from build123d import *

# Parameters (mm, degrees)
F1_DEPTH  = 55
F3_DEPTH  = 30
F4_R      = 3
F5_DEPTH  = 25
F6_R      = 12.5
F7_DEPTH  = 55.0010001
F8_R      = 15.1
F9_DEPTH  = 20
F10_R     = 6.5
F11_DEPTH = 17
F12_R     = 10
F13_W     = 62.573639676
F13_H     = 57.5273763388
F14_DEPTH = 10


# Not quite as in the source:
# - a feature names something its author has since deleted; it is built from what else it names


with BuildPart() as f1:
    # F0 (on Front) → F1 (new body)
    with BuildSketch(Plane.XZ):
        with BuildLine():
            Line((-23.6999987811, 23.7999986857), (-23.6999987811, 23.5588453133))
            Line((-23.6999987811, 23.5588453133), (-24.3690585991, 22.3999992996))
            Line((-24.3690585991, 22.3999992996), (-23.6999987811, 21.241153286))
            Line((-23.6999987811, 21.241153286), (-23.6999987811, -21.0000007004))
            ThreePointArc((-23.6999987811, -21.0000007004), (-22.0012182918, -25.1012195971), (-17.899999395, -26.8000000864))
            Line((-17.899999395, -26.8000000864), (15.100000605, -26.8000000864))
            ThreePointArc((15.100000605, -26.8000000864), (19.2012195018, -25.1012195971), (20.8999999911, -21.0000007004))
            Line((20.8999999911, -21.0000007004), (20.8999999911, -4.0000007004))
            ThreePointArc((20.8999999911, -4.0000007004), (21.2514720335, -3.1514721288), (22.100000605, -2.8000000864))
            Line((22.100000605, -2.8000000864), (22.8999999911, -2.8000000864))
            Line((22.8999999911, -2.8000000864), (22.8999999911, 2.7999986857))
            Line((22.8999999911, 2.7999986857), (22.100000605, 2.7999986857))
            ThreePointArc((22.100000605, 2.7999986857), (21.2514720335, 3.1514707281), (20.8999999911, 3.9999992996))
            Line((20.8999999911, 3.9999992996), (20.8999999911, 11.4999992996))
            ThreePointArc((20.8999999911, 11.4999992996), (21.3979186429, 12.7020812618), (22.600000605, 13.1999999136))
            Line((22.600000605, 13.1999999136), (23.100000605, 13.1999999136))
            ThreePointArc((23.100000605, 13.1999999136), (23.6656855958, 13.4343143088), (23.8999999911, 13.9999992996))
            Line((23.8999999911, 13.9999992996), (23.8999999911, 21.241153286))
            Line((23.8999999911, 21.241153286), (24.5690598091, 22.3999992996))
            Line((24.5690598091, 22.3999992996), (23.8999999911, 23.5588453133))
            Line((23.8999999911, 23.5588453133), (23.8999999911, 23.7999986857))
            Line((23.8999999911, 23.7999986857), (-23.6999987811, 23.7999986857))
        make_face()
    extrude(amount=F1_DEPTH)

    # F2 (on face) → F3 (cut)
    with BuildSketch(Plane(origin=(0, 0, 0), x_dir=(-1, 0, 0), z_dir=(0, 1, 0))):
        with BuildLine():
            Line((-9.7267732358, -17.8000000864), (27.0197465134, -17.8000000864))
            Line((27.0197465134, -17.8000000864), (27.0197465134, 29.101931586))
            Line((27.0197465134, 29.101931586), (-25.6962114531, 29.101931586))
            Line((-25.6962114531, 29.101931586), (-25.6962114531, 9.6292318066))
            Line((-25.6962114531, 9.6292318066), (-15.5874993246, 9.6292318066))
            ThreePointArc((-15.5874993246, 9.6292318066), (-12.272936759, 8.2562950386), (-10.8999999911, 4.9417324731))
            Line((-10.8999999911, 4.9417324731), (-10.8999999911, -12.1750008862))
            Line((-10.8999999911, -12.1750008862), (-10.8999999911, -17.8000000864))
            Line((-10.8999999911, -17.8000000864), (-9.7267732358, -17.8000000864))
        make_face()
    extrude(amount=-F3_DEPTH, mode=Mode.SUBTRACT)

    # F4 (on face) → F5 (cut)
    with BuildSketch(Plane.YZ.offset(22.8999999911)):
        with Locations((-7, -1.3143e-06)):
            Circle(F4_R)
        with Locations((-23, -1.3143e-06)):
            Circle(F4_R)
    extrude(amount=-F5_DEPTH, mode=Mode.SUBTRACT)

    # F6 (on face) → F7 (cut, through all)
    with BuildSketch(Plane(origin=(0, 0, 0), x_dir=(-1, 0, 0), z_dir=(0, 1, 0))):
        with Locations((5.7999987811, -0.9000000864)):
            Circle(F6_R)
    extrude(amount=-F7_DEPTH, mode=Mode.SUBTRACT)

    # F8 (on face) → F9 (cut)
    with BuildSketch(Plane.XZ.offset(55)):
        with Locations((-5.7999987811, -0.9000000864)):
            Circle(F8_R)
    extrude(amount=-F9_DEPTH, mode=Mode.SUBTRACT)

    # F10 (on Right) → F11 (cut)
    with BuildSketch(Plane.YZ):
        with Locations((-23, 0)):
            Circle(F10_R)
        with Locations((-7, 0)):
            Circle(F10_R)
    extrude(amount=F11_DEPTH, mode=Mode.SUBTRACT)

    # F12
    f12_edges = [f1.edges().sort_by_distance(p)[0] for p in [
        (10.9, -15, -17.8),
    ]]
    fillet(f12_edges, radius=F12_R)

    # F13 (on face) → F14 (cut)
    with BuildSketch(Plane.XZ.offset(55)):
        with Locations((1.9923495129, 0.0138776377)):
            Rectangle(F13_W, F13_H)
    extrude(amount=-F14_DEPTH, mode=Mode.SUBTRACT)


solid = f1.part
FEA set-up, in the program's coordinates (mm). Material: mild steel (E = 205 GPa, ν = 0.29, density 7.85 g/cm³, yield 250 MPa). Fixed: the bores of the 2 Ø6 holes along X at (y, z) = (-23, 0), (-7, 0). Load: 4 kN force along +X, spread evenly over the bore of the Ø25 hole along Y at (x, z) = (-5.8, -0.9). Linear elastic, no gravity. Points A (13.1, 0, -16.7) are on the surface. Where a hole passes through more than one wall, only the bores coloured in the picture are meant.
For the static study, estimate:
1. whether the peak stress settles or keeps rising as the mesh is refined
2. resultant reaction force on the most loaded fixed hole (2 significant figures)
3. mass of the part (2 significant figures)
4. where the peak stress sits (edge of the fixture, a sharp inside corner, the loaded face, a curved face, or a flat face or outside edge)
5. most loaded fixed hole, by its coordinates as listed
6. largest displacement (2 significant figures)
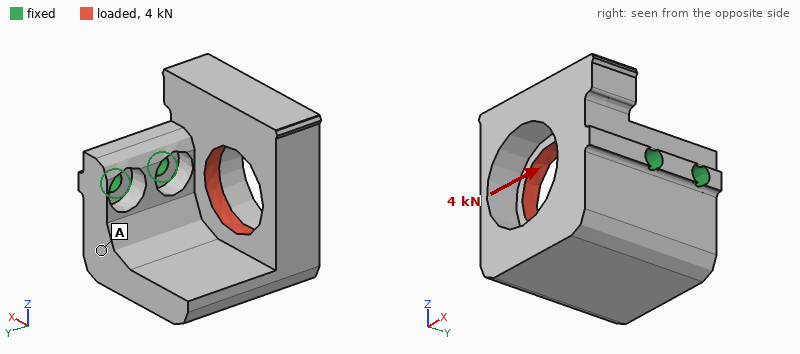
keeps rising
5.1 kN
340 g
edge of the fixture
(-23, 0)
33 µm
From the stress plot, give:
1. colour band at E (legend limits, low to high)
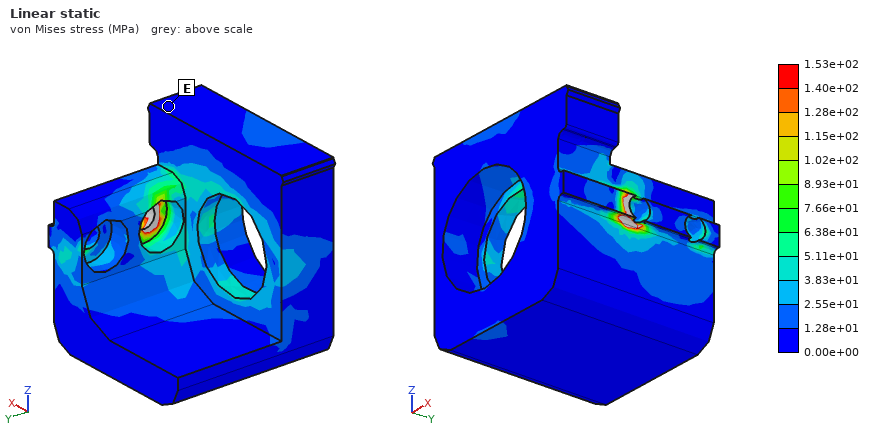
0.00e+00 to 1.28e+01 MPa
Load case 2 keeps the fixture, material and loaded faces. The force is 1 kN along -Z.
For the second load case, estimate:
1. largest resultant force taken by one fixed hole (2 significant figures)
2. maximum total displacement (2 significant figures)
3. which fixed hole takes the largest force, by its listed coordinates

1.3 kN
55 µm
(-23, 0)
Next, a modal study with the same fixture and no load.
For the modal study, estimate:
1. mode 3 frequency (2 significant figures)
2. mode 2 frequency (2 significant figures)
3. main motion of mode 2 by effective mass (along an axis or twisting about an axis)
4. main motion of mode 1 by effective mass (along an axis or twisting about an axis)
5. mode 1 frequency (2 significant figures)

4900 Hz
2600 Hz
along Y
along Z
1500 Hz
